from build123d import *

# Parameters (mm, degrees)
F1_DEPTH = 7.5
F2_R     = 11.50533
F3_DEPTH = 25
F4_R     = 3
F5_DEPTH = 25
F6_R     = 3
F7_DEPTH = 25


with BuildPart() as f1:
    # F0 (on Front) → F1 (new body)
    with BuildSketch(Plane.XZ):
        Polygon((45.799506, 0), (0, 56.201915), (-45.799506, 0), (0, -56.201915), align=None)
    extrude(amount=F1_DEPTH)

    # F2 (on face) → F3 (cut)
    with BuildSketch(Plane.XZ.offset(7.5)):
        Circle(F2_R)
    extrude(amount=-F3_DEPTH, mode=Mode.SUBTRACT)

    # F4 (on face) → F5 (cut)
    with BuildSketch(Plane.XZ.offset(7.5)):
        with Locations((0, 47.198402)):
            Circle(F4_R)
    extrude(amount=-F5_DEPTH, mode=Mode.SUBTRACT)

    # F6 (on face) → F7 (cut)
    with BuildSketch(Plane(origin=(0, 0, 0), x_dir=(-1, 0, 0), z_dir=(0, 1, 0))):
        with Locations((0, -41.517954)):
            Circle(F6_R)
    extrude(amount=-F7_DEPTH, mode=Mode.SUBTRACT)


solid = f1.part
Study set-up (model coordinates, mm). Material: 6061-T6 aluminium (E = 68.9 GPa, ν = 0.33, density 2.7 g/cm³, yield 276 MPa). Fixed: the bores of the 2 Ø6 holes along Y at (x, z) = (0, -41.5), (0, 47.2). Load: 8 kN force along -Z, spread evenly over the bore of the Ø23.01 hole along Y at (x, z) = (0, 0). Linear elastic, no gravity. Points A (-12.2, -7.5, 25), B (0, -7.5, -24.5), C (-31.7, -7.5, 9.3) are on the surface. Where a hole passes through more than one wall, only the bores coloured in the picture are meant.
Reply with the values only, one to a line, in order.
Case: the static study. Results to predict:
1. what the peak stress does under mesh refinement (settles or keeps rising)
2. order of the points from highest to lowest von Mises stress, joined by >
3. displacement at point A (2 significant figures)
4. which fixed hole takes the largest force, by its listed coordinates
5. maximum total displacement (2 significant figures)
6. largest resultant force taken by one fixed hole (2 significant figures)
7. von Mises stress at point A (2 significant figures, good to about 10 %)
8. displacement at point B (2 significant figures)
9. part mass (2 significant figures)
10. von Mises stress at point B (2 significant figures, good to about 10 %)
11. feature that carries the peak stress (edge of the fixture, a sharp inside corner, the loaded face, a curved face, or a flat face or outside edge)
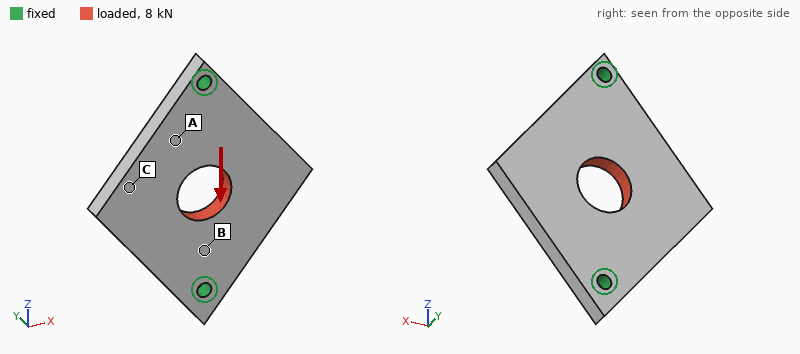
keeps rising
B > A > C
8.3 µm
(0, -41.5)
13 µm
4.2 kN
13 MPa
6.2 µm
95 g
23 MPa
edge of the fixture
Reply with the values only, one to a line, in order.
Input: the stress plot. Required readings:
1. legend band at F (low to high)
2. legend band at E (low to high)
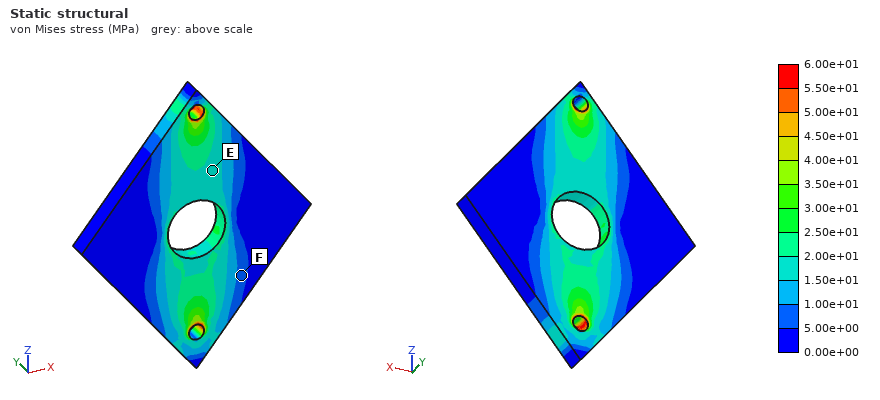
5.00e+00 to 1.00e+01 MPa
1.50e+01 to 2.00e+01 MPa
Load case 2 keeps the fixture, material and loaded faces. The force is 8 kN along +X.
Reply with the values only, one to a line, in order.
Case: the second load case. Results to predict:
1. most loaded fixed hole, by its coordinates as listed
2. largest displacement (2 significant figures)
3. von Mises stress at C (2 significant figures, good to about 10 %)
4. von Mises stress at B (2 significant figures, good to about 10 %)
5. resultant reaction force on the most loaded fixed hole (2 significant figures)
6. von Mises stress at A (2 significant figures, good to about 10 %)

(0, -41.5)
30 µm
16 MPa
17 MPa
4.2 kN
18 MPa
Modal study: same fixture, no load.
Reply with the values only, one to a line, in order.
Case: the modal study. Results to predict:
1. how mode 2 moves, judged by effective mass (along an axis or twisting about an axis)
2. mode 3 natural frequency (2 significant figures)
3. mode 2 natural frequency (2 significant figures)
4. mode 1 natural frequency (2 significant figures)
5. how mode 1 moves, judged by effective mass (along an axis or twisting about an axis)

along Y
8000 Hz
3000 Hz
2400 Hz
twisting about Z
